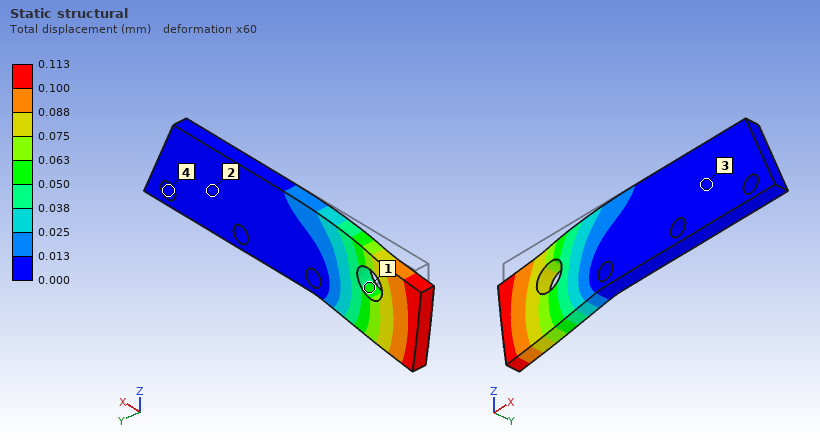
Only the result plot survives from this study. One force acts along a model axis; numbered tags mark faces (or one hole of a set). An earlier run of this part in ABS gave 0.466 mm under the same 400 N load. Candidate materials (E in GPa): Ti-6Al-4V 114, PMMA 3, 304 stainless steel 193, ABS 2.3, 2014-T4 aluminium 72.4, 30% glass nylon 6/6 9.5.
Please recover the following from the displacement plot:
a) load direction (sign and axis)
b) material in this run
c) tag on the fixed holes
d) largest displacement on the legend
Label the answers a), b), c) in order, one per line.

a) -Z
b) 30% glass nylon 6/6
c) 4
d) 0.113 mm
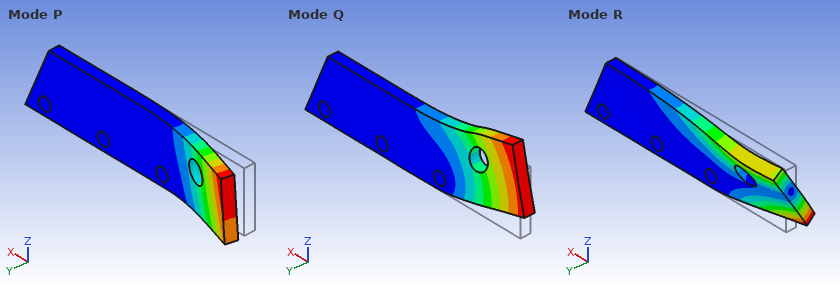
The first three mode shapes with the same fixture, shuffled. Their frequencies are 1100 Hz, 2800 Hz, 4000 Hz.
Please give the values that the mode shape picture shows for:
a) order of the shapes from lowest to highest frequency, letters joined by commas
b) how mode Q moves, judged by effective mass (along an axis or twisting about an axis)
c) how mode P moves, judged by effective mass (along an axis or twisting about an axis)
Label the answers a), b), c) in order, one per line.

a) P, R, Q
b) along Z
c) along Y
